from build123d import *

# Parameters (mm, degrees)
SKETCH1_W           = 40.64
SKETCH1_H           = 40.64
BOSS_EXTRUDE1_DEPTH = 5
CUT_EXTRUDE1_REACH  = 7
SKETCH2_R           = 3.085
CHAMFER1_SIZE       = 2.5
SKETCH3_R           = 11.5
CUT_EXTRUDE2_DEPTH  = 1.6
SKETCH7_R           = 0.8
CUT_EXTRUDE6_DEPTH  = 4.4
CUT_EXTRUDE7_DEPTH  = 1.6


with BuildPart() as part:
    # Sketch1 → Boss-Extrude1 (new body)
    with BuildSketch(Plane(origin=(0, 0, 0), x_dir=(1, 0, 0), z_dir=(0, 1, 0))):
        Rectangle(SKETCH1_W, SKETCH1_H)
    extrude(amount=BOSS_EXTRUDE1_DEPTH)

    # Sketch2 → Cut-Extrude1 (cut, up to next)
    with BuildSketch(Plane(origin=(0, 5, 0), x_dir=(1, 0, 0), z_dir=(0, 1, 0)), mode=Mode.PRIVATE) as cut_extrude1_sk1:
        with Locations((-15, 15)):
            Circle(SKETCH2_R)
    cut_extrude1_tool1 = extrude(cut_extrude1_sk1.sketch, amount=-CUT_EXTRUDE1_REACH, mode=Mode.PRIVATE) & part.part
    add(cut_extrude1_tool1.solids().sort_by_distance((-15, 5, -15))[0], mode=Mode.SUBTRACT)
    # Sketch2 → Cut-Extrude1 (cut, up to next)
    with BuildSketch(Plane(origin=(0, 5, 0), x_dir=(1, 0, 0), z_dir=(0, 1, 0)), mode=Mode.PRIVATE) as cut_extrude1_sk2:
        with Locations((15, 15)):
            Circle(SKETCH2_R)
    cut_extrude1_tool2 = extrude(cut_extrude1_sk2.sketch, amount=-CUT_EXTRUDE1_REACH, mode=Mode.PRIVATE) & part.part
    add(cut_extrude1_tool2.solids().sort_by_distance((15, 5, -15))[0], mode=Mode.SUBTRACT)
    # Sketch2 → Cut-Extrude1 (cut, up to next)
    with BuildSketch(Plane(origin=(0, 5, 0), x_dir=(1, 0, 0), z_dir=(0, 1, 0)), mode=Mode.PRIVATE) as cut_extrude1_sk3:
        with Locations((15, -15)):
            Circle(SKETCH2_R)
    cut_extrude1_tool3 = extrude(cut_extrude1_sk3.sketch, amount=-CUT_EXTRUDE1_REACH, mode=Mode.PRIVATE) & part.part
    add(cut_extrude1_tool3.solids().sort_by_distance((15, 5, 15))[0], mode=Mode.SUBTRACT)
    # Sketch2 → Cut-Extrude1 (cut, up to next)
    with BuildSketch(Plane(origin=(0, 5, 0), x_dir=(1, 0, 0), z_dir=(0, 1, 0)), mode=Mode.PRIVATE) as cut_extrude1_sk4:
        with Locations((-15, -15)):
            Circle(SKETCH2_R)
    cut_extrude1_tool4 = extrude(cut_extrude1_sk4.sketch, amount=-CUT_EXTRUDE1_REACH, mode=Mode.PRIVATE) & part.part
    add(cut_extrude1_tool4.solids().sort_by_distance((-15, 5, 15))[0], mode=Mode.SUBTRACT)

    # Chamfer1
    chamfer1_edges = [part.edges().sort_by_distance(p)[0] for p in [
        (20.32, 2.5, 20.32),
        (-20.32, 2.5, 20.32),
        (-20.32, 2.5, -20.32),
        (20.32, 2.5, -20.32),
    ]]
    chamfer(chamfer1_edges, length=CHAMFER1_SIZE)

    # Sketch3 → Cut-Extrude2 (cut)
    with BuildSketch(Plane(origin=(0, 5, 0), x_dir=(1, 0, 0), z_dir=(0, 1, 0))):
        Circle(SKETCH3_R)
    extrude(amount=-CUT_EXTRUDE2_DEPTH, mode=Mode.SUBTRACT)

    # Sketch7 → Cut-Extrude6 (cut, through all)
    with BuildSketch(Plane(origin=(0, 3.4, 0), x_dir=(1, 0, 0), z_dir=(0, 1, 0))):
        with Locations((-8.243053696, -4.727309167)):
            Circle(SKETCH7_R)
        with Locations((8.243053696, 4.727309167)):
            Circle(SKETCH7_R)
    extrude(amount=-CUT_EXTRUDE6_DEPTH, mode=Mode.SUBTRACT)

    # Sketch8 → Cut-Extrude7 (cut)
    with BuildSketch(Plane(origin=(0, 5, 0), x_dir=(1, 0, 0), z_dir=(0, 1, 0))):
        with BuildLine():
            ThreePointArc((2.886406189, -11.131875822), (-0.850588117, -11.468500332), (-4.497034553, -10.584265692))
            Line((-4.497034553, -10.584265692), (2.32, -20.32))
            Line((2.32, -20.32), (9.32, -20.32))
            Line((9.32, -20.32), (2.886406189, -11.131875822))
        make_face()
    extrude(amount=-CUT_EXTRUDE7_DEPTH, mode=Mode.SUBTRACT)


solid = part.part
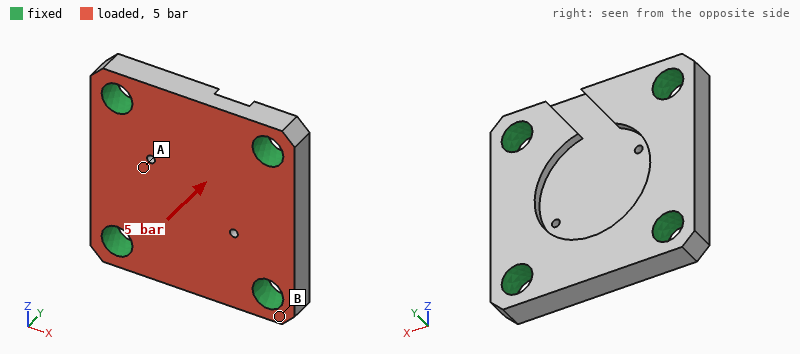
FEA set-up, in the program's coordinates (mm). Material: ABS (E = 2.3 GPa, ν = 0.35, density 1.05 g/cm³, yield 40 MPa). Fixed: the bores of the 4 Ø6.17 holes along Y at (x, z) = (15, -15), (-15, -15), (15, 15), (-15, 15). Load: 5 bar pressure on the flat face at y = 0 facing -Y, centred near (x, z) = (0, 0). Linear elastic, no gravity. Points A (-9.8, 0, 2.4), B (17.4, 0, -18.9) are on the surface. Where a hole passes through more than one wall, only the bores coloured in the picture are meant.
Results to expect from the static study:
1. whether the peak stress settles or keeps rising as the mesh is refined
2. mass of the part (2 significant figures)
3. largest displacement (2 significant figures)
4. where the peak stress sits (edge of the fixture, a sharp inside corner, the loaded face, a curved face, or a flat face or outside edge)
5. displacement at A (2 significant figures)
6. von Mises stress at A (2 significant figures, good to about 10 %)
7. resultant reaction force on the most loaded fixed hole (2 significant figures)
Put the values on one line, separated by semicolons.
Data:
keeps rising; 7.2 g; 0.12 mm; edge of the fixture; 0.072 mm; 4.3 MPa; 200 N
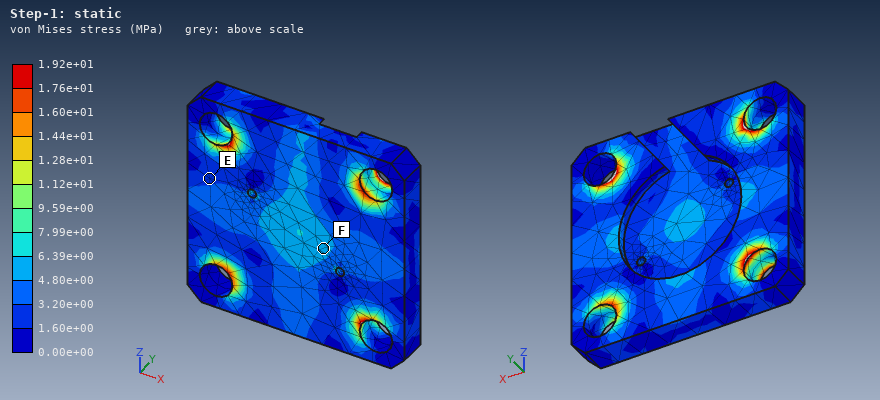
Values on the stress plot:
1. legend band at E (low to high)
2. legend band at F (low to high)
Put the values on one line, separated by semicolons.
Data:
1.60e+00 to 3.20e+00 MPa; 4.80e+00 to 6.39e+00 MPa
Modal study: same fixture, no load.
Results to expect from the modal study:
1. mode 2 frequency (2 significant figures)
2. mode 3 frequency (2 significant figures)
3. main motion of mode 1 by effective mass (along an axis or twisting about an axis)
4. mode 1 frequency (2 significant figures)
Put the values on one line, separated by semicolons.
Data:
9600 Hz; 9700 Hz; along Y; 6600 Hz
